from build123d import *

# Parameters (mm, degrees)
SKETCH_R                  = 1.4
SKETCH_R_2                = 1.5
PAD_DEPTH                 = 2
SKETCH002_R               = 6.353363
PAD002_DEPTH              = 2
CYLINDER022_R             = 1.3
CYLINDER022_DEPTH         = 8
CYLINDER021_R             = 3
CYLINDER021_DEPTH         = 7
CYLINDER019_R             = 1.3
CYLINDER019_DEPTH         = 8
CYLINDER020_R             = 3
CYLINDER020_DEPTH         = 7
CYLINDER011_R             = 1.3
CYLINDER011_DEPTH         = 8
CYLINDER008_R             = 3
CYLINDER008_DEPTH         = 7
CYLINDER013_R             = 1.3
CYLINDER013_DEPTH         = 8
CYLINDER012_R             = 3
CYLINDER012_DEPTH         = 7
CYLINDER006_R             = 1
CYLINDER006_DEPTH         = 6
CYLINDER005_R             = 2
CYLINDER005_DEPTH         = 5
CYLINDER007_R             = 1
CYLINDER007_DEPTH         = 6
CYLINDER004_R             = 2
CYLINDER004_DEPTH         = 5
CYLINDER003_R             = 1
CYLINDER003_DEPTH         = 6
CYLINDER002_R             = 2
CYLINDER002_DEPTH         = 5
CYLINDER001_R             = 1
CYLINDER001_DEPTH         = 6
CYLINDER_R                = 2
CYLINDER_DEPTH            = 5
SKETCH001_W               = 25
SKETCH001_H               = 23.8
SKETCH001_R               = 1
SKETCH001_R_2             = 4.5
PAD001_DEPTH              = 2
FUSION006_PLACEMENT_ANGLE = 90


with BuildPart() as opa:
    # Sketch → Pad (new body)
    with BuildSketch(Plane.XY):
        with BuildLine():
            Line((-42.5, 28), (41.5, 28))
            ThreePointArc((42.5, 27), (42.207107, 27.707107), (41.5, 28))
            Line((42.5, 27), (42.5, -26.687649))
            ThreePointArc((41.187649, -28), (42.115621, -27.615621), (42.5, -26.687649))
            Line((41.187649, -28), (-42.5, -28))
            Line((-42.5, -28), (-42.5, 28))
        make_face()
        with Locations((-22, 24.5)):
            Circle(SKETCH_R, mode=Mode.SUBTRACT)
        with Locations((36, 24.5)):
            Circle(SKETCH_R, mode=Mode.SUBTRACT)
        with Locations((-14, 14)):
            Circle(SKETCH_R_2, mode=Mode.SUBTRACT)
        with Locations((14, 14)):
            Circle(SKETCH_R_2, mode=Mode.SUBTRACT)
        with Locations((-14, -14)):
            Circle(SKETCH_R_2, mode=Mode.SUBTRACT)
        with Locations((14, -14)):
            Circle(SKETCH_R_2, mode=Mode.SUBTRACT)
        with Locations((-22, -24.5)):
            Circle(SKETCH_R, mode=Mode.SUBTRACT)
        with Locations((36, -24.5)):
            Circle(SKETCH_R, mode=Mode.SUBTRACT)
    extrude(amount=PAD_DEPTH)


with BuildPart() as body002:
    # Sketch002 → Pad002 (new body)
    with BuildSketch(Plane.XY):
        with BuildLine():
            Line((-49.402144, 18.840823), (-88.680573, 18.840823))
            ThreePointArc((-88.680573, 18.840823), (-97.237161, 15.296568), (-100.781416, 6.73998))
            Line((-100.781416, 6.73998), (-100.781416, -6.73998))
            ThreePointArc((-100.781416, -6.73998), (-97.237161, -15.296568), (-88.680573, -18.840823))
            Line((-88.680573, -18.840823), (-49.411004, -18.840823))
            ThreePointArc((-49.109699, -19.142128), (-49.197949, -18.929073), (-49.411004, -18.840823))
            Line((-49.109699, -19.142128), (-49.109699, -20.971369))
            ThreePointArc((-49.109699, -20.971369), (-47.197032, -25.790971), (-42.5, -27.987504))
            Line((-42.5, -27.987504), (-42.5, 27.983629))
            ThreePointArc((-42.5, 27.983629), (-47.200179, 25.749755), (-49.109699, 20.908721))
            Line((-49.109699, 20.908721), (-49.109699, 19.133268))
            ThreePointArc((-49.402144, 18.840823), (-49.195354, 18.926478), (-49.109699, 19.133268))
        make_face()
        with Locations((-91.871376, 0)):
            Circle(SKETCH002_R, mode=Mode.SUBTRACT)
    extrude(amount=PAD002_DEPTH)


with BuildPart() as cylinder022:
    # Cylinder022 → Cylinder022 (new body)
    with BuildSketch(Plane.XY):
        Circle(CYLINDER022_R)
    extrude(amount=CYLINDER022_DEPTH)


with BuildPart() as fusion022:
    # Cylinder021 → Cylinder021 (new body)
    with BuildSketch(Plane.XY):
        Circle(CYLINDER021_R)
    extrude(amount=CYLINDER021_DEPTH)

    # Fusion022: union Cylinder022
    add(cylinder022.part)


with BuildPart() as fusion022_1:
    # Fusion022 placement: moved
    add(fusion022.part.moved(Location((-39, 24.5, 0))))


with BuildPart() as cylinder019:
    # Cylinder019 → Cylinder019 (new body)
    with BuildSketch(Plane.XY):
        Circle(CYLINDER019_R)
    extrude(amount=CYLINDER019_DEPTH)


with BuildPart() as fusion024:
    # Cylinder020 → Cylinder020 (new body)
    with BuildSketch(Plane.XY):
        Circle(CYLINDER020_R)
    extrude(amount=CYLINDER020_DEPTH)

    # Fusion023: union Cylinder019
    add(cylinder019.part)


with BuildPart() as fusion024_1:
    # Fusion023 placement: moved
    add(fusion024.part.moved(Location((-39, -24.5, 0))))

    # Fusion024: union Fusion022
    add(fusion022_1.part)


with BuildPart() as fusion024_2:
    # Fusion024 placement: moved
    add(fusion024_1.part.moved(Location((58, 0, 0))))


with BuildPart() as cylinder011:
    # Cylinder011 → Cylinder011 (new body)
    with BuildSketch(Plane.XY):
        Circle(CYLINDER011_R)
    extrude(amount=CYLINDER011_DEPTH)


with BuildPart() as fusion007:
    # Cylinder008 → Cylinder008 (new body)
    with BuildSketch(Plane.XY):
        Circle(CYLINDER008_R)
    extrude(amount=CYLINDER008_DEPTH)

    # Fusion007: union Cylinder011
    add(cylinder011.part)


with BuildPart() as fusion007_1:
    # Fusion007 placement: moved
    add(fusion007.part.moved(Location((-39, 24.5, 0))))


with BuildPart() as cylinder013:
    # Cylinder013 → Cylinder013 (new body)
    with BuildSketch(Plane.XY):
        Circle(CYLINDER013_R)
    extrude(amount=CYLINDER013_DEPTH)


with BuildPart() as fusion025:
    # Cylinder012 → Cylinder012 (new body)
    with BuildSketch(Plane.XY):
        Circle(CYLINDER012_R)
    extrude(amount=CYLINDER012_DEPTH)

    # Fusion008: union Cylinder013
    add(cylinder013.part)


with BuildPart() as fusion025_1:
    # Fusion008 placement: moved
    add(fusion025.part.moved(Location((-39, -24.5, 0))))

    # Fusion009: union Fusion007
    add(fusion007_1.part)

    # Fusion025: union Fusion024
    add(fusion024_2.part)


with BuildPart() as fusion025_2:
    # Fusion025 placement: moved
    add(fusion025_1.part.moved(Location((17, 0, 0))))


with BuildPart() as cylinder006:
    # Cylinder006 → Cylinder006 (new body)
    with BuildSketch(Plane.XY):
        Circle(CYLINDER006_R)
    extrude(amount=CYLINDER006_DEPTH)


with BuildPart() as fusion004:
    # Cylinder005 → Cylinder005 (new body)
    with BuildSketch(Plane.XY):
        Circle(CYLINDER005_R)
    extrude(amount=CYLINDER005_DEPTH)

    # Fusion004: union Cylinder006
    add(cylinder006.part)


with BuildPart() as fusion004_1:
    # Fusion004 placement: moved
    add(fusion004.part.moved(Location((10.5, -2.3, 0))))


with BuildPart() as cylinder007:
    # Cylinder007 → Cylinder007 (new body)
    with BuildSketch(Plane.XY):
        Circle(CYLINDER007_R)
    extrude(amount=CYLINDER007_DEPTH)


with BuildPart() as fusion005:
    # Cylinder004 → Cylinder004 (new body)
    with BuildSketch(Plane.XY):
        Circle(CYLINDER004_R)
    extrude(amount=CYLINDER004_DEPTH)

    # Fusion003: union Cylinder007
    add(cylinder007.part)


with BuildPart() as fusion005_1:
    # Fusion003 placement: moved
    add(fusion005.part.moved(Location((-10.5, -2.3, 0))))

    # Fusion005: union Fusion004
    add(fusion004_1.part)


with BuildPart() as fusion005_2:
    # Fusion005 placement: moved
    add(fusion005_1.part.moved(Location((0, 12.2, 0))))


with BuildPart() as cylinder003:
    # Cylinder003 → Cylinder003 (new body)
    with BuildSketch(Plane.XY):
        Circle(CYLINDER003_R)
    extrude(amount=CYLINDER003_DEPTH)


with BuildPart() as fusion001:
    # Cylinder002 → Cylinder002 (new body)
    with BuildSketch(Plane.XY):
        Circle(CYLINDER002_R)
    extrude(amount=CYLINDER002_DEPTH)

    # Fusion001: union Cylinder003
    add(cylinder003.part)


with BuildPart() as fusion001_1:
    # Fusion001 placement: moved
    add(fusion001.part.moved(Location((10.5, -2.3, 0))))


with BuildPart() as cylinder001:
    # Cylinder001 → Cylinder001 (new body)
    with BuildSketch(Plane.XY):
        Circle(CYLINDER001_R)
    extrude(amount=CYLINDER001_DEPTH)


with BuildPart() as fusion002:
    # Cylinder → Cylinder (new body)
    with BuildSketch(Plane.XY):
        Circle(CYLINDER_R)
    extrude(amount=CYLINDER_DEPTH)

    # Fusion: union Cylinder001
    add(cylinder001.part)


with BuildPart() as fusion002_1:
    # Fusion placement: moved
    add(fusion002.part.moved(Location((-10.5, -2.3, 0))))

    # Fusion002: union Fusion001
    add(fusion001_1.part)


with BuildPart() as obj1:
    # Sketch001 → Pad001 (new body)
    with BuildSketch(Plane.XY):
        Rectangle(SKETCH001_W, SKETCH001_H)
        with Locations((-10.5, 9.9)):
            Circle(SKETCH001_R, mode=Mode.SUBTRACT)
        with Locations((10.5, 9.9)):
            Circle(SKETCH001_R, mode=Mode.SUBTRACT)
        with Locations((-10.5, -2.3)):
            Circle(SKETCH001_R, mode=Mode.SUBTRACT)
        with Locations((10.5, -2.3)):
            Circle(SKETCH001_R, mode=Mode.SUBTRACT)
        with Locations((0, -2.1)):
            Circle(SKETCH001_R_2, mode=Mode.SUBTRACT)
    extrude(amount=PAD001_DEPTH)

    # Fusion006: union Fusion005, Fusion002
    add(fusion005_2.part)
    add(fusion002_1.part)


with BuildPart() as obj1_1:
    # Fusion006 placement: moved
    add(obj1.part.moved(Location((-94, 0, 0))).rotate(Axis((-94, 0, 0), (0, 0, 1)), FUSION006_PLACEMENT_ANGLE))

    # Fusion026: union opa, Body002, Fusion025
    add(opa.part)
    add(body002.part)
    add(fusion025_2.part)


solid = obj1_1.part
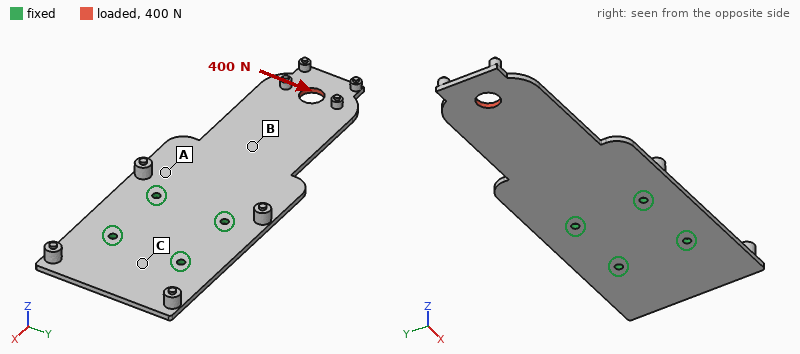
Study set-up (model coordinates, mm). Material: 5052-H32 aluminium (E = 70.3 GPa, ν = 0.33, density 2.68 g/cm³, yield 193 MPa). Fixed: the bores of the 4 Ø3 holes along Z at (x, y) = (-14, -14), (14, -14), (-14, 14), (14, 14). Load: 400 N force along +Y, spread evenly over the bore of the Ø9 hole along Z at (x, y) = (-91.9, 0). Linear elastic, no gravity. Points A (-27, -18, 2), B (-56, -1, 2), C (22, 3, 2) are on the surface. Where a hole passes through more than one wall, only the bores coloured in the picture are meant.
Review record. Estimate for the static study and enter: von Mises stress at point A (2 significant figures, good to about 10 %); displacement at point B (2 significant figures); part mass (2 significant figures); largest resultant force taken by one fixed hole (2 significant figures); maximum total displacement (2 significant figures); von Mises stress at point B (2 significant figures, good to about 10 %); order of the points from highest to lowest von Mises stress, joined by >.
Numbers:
19 MPa
26 µm
40 g
730 N
96 µm
11 MPa
A > B > C
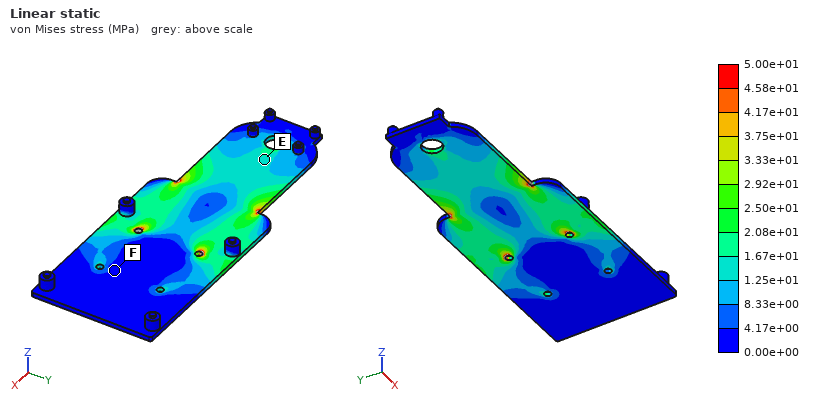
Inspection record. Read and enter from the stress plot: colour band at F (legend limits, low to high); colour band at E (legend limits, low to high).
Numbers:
0.00e+00 to 4.17e+00 MPa
1.25e+01 to 1.67e+01 MPa
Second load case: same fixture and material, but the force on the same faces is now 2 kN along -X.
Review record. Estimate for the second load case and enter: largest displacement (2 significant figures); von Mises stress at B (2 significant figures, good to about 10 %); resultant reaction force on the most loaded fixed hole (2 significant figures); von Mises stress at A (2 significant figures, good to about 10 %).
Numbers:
38 µm
24 MPa
790 N
19 MPa
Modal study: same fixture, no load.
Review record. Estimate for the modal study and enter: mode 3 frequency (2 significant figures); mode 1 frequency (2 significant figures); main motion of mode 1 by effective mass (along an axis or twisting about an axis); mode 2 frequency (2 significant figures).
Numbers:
1300 Hz
240 Hz
along Z
1100 Hz
